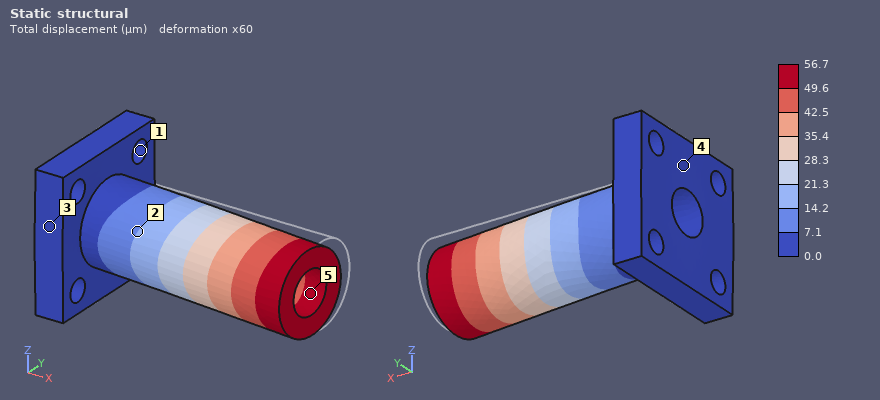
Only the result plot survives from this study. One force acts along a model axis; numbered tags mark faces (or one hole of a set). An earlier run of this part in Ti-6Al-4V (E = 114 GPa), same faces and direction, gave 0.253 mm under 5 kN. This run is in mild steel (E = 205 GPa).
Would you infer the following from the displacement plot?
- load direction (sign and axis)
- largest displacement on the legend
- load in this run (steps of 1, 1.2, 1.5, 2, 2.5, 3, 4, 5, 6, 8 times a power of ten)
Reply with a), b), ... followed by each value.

a) -Y
b) 56.7 µm
c) 2 kN
